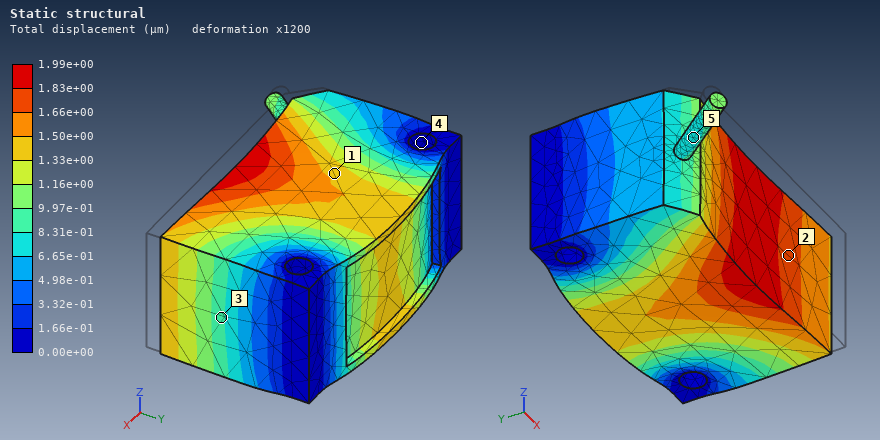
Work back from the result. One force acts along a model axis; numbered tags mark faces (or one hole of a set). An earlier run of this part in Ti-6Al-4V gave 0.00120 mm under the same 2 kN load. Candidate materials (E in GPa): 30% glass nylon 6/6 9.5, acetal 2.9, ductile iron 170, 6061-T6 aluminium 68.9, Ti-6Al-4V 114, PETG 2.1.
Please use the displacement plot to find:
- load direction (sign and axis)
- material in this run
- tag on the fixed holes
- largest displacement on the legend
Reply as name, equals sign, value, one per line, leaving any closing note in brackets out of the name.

load direction = +Y
material in this run = 6061-T6 aluminium
tag on the fixed holes = 4
largest displacement on the legend = 1.99e+00 µm
